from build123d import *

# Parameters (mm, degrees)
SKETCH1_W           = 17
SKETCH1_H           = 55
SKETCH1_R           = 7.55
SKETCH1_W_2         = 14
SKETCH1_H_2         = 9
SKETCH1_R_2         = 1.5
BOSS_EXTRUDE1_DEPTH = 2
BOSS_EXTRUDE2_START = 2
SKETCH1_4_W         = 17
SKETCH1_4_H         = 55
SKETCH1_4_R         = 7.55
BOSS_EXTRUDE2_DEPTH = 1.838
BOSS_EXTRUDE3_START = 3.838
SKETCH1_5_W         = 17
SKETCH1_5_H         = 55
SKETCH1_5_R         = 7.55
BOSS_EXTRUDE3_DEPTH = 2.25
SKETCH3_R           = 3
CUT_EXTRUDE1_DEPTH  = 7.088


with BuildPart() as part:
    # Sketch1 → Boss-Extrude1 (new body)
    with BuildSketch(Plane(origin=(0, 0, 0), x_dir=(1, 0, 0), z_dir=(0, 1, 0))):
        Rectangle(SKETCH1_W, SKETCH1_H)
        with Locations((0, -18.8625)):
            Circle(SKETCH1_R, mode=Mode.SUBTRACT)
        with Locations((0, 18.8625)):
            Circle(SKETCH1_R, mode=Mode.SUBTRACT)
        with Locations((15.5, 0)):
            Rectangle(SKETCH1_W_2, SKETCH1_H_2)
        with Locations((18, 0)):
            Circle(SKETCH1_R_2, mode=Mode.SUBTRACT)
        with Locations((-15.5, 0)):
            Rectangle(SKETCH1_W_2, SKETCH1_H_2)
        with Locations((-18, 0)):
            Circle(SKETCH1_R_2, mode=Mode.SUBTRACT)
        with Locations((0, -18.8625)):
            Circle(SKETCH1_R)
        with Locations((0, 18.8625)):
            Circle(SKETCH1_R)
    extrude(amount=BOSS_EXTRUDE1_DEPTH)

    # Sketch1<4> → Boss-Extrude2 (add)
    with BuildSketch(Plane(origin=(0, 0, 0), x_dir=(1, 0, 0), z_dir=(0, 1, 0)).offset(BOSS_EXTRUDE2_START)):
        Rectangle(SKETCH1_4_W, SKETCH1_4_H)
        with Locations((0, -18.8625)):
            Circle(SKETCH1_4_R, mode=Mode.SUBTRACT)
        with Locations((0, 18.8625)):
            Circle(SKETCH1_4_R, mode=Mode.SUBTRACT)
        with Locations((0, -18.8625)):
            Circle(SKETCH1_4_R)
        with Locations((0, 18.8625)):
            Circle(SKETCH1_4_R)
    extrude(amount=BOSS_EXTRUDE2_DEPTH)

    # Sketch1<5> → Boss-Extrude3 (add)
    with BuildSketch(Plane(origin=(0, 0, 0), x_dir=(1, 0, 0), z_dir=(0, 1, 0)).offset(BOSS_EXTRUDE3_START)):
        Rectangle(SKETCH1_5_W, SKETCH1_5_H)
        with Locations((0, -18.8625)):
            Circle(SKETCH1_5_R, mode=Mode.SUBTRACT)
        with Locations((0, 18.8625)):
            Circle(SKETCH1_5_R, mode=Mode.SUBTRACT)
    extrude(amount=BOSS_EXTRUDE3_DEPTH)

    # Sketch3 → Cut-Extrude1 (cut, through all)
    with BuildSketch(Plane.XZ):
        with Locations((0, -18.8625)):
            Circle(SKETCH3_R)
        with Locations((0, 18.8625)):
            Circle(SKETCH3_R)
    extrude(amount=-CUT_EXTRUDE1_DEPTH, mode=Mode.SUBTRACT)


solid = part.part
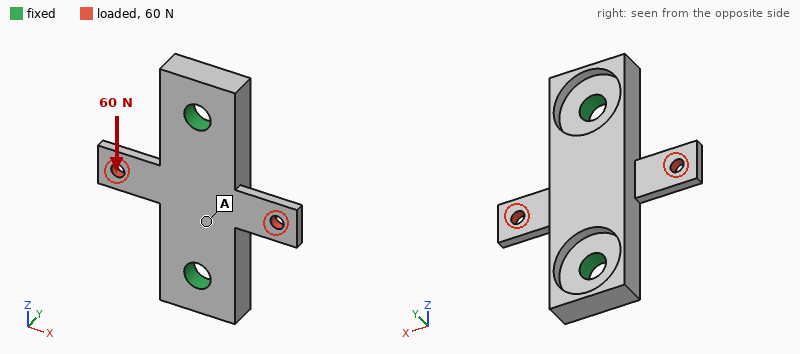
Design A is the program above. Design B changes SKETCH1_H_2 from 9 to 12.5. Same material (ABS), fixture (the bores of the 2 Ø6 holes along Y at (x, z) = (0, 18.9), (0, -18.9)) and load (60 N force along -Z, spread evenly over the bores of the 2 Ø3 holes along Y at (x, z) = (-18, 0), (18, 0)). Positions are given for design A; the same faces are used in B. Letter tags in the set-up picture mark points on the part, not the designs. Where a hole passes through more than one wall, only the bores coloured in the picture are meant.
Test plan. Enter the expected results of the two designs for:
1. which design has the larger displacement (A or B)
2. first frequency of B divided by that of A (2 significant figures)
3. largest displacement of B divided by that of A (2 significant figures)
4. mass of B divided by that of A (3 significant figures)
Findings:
A
0.96
0.50
1.04
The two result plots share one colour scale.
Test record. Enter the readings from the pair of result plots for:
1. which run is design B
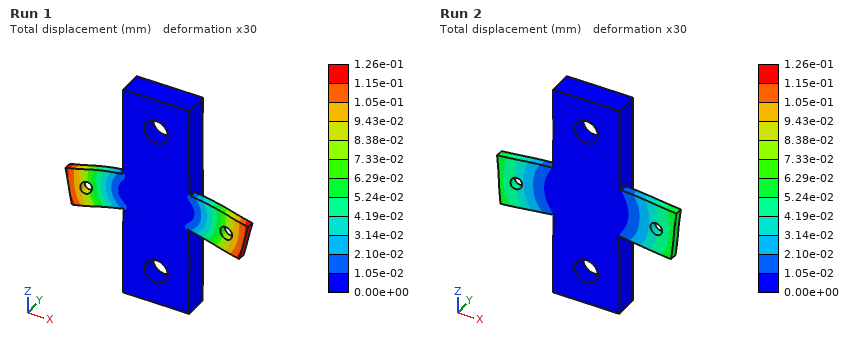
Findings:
Run 2
